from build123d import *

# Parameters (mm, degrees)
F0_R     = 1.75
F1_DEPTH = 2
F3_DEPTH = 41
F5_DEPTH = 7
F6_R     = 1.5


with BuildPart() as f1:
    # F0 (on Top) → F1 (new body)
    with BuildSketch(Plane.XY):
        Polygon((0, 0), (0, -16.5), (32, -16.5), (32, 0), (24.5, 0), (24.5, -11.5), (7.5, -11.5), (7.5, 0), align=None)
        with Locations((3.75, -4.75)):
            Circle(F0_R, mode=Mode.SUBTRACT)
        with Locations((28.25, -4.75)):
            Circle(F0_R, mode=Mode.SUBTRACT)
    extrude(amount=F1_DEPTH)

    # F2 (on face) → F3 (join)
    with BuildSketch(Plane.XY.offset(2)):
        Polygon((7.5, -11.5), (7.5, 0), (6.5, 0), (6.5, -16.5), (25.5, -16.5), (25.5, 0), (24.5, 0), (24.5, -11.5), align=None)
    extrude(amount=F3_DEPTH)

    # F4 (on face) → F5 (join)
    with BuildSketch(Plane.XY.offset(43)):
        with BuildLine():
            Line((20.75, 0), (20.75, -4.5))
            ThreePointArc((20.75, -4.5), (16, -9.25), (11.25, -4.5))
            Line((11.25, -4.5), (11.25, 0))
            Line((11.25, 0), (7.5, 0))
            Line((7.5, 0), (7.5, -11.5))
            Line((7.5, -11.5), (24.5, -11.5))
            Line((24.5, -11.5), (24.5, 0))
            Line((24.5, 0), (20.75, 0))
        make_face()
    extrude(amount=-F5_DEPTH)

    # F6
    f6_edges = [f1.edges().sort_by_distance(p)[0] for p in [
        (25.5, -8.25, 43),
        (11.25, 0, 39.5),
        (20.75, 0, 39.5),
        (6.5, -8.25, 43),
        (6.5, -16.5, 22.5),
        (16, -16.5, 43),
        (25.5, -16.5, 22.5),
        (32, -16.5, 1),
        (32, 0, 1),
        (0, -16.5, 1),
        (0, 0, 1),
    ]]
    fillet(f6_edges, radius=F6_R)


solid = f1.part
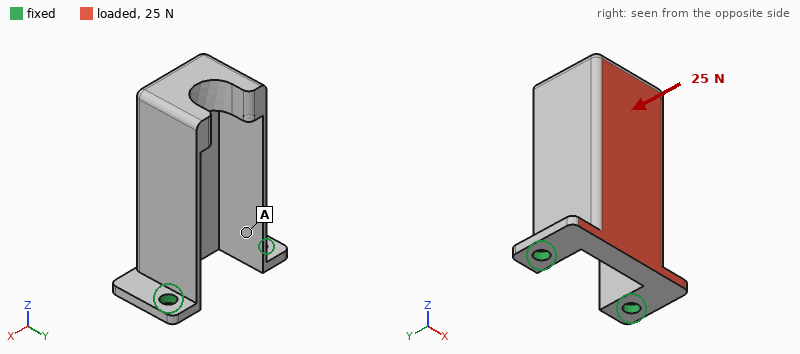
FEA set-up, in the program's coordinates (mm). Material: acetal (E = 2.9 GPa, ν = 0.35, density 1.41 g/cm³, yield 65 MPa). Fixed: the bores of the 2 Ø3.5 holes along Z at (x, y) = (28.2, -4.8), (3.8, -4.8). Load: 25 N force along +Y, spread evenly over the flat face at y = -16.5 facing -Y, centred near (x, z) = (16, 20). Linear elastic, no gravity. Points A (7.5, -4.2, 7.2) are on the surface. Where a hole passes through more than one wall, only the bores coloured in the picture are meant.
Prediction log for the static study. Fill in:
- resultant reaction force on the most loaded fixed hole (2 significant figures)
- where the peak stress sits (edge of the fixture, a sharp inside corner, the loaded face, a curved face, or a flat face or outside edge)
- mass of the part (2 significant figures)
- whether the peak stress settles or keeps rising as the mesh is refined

13 N
edge of the fixture
8.8 g
keeps rising
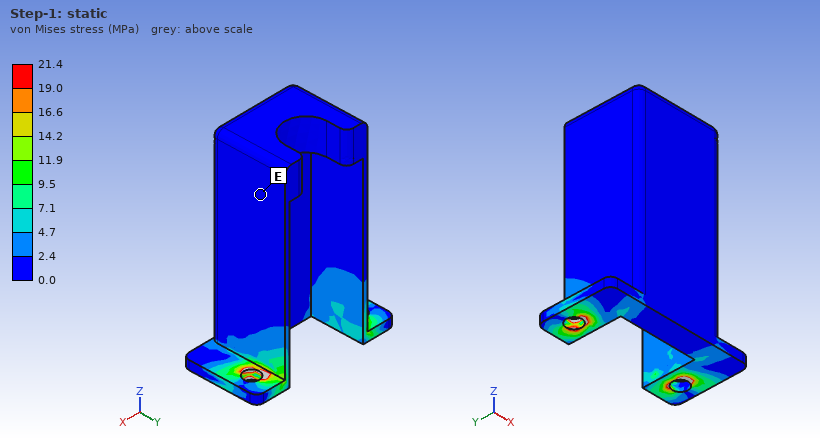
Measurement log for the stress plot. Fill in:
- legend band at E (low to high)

0.0 to 2.4 MPa
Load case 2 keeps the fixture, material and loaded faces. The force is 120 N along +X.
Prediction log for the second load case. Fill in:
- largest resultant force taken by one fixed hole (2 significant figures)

130 N
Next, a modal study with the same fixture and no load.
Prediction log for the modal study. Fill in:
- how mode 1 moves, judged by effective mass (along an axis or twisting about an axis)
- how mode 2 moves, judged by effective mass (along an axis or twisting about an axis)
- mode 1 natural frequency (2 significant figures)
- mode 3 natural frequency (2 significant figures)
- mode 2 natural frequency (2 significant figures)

along Y
along X
350 Hz
2100 Hz
720 Hz
